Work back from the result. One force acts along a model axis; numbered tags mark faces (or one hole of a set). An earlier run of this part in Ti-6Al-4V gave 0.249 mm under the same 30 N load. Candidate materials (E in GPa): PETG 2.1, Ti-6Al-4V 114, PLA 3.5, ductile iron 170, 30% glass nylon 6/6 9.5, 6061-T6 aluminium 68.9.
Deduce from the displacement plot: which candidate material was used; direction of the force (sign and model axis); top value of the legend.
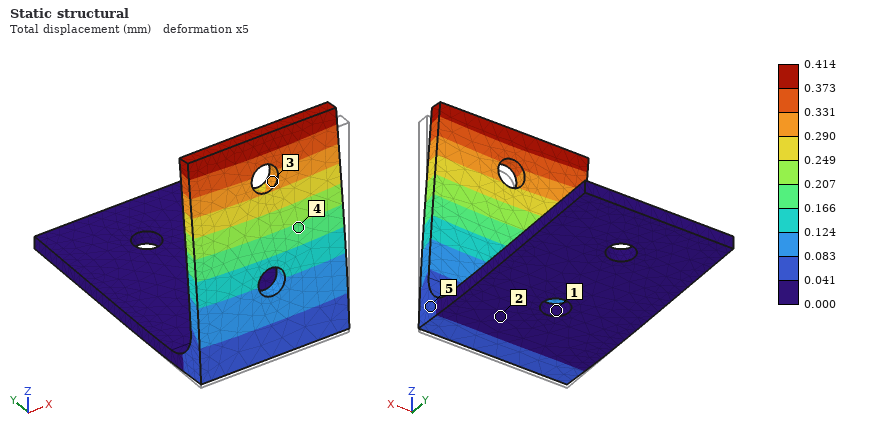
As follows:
6061-T6 aluminium
+Y
0.414 mm
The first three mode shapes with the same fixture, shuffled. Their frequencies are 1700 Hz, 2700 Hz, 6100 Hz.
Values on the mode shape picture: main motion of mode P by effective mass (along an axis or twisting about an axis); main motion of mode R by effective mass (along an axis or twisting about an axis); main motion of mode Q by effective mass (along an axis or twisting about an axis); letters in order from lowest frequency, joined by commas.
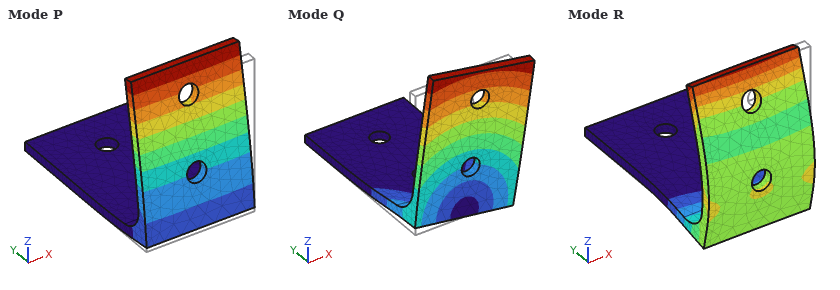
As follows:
along Y
along Z
along X
P, Q, R
